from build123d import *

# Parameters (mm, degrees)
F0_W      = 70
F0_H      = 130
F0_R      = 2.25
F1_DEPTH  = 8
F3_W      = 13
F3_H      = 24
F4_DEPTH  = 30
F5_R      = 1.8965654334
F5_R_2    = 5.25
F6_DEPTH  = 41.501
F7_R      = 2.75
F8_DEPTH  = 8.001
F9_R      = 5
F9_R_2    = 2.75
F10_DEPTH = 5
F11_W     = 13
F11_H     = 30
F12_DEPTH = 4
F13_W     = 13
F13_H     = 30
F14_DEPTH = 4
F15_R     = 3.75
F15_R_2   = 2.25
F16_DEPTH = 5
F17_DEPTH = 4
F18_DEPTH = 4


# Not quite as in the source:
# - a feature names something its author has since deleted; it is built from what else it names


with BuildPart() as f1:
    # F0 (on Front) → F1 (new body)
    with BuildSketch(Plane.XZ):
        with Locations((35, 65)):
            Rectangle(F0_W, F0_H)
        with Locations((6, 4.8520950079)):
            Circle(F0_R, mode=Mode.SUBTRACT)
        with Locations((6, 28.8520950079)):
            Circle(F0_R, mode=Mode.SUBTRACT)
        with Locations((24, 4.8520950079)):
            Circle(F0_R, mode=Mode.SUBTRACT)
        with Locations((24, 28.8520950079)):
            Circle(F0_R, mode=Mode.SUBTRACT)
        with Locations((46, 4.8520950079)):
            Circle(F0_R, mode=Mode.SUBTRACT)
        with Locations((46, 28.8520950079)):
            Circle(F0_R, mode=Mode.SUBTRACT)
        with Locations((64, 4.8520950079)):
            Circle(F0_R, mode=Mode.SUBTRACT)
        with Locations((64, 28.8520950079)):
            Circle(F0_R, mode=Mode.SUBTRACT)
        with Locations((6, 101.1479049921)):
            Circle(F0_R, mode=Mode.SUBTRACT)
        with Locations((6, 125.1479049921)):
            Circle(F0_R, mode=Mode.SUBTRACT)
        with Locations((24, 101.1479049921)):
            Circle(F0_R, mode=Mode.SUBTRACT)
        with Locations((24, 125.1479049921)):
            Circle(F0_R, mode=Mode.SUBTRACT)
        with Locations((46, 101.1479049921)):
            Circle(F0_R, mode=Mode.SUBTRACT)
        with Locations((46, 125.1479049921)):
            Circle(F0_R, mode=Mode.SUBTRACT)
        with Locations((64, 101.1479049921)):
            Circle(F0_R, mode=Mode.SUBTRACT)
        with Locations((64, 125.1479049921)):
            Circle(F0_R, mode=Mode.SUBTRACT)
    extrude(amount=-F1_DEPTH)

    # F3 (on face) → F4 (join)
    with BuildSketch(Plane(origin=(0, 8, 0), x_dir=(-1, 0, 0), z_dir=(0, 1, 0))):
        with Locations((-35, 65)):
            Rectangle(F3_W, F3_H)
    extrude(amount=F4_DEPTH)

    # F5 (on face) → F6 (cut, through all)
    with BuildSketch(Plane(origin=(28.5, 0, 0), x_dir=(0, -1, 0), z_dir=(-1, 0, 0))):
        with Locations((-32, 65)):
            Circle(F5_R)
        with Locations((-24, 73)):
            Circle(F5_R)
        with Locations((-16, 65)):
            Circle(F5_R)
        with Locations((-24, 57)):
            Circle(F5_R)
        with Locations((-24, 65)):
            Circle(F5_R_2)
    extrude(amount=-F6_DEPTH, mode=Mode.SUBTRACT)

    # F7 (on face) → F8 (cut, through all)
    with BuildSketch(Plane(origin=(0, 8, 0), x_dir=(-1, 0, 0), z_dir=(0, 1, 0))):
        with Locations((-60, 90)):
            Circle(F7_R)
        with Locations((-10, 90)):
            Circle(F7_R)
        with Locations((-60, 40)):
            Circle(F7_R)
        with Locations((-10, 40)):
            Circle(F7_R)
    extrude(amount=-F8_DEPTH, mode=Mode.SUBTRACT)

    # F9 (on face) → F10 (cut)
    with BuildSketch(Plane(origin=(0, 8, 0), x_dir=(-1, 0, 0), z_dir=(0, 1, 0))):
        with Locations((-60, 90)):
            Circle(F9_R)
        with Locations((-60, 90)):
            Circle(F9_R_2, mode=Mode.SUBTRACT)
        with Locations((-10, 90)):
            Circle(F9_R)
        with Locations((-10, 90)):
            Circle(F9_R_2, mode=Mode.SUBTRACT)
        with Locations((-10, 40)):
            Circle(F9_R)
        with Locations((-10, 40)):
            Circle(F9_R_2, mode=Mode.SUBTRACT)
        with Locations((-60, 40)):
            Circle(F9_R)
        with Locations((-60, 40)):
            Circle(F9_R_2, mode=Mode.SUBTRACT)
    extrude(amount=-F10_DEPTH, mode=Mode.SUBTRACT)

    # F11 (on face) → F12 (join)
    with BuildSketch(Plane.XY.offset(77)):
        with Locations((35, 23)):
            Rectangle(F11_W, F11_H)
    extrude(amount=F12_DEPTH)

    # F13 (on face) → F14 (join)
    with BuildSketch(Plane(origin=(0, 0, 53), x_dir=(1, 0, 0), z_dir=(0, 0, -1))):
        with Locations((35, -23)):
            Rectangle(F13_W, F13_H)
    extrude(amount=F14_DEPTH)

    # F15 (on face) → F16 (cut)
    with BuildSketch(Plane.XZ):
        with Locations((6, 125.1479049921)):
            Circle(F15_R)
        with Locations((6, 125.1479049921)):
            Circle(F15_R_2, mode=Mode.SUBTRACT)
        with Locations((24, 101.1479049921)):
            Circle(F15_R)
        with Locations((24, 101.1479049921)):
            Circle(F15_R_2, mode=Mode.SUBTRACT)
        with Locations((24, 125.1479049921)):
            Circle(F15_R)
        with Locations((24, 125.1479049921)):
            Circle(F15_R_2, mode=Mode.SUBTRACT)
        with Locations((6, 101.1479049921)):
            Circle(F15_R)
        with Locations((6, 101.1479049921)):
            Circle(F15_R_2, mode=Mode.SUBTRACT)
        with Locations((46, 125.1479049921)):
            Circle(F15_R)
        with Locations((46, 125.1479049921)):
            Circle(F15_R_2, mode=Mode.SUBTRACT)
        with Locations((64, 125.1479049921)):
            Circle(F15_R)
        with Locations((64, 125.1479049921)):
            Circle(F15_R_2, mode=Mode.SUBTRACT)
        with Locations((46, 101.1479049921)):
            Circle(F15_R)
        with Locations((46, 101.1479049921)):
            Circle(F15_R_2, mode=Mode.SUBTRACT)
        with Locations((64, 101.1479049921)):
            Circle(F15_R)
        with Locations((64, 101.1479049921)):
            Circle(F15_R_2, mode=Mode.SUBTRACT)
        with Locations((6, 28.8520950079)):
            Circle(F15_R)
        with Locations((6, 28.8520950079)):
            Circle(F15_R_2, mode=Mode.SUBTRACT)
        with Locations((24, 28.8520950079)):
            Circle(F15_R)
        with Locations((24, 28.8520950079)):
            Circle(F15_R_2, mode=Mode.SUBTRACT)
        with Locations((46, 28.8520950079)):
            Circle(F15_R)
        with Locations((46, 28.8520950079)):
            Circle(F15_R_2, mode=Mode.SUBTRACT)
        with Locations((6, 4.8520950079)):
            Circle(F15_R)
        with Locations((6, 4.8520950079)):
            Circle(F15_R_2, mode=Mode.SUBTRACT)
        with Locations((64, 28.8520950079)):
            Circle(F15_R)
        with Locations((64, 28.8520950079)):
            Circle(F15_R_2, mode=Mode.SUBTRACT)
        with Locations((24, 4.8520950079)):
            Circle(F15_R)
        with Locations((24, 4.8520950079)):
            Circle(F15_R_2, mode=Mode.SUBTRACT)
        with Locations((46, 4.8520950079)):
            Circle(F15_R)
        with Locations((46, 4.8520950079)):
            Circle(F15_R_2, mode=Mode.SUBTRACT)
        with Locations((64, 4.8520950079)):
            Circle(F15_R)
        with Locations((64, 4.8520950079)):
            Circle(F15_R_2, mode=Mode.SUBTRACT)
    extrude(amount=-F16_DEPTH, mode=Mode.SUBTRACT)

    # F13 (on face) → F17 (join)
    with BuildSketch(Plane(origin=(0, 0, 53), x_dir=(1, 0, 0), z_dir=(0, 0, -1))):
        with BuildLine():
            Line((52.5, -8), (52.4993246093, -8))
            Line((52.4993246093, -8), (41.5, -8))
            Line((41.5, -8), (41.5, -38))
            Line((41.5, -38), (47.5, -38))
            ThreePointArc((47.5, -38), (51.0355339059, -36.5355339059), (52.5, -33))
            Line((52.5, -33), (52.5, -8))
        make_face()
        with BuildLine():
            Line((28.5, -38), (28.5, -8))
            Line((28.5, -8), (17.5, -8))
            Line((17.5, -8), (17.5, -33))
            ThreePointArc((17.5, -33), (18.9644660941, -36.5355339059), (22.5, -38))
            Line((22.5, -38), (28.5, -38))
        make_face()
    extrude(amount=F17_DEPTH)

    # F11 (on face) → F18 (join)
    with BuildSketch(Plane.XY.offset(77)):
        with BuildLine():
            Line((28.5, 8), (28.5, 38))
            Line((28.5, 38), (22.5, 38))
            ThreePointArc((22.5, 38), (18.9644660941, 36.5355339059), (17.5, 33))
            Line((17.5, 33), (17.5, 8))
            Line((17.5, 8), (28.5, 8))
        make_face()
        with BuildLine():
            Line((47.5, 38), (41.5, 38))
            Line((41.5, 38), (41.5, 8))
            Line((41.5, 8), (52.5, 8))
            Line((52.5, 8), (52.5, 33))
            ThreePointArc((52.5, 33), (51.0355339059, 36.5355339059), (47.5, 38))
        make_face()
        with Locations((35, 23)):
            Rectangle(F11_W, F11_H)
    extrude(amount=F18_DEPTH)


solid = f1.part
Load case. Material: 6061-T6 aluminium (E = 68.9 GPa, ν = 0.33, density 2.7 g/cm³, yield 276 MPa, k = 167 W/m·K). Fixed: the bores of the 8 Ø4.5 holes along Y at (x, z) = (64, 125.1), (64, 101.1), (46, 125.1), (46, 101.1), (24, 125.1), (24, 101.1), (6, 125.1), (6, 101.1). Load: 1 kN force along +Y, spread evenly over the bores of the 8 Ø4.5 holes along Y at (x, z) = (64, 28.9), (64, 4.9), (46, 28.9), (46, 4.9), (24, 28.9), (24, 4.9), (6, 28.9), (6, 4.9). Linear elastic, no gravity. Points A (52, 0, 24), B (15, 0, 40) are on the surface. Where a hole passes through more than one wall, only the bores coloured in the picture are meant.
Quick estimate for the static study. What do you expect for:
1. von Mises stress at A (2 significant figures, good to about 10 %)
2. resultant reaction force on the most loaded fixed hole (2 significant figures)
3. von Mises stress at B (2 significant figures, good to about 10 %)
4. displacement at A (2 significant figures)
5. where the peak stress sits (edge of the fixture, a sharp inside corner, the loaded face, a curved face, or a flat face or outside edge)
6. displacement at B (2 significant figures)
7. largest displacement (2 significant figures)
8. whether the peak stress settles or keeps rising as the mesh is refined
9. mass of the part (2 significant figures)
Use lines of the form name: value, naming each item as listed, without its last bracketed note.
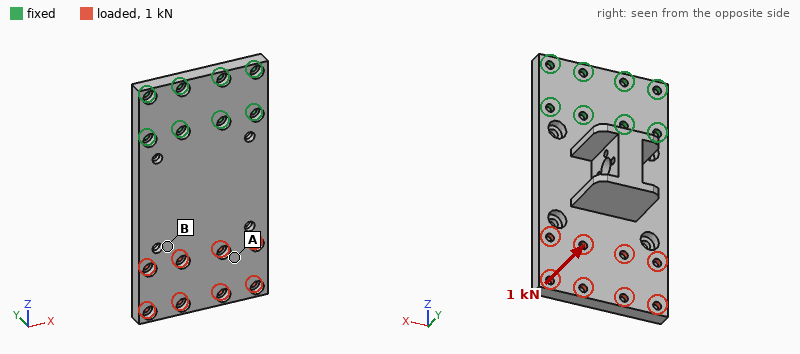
von Mises stress at A: 16 MPa
resultant reaction force on the most loaded fixed hole: 2.5 kN
von Mises stress at B: 37 MPa
displacement at A: 0.96 mm
where the peak stress sits: edge of the fixture
displacement at B: 0.70 mm
largest displacement: 1.4 mm
whether the peak stress settles or keeps rising as the mesh is refined: keeps rising
mass of the part: 220 g
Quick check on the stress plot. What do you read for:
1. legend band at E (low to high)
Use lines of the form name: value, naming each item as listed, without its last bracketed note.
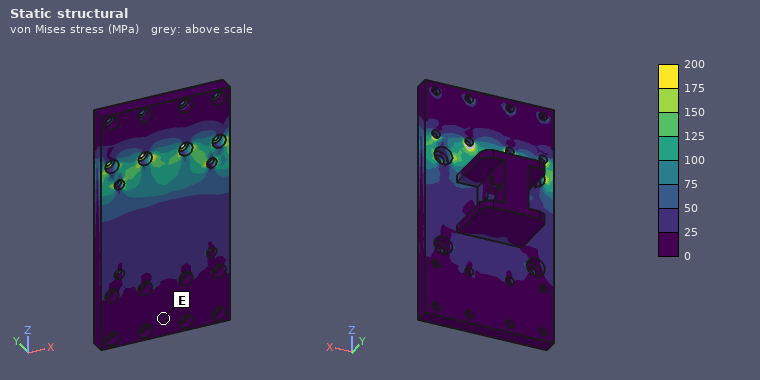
legend band at E: 0 to 25 MPa
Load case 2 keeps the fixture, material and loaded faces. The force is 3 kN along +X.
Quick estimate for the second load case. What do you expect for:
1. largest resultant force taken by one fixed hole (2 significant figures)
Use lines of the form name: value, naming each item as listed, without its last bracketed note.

largest resultant force taken by one fixed hole: 2.7 kN
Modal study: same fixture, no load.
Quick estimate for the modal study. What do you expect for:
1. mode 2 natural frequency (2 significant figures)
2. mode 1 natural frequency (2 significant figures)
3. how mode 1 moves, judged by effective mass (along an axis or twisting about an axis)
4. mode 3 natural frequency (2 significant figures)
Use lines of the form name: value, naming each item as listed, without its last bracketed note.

mode 2 natural frequency: 2200 Hz
mode 1 natural frequency: 590 Hz
how mode 1 moves, judged by effective mass: along Y
mode 3 natural frequency: 3300 Hz
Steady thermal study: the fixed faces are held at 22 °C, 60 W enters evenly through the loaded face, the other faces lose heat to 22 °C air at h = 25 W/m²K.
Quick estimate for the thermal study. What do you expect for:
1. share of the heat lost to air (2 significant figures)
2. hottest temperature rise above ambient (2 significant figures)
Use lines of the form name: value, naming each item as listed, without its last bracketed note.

share of the heat lost to air: 26 %
hottest temperature rise above ambient: 53 K
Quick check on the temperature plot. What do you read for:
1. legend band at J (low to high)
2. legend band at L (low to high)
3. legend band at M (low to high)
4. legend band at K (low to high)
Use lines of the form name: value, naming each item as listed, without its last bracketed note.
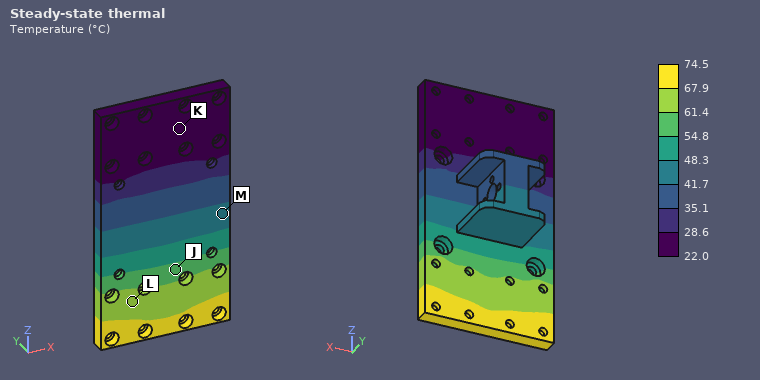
legend band at J: 54.8 to 61.4 °C
legend band at L: 61.4 to 67.9 °C
legend band at M: 41.7 to 48.3 °C
legend band at K: 22.0 to 28.6 °C
